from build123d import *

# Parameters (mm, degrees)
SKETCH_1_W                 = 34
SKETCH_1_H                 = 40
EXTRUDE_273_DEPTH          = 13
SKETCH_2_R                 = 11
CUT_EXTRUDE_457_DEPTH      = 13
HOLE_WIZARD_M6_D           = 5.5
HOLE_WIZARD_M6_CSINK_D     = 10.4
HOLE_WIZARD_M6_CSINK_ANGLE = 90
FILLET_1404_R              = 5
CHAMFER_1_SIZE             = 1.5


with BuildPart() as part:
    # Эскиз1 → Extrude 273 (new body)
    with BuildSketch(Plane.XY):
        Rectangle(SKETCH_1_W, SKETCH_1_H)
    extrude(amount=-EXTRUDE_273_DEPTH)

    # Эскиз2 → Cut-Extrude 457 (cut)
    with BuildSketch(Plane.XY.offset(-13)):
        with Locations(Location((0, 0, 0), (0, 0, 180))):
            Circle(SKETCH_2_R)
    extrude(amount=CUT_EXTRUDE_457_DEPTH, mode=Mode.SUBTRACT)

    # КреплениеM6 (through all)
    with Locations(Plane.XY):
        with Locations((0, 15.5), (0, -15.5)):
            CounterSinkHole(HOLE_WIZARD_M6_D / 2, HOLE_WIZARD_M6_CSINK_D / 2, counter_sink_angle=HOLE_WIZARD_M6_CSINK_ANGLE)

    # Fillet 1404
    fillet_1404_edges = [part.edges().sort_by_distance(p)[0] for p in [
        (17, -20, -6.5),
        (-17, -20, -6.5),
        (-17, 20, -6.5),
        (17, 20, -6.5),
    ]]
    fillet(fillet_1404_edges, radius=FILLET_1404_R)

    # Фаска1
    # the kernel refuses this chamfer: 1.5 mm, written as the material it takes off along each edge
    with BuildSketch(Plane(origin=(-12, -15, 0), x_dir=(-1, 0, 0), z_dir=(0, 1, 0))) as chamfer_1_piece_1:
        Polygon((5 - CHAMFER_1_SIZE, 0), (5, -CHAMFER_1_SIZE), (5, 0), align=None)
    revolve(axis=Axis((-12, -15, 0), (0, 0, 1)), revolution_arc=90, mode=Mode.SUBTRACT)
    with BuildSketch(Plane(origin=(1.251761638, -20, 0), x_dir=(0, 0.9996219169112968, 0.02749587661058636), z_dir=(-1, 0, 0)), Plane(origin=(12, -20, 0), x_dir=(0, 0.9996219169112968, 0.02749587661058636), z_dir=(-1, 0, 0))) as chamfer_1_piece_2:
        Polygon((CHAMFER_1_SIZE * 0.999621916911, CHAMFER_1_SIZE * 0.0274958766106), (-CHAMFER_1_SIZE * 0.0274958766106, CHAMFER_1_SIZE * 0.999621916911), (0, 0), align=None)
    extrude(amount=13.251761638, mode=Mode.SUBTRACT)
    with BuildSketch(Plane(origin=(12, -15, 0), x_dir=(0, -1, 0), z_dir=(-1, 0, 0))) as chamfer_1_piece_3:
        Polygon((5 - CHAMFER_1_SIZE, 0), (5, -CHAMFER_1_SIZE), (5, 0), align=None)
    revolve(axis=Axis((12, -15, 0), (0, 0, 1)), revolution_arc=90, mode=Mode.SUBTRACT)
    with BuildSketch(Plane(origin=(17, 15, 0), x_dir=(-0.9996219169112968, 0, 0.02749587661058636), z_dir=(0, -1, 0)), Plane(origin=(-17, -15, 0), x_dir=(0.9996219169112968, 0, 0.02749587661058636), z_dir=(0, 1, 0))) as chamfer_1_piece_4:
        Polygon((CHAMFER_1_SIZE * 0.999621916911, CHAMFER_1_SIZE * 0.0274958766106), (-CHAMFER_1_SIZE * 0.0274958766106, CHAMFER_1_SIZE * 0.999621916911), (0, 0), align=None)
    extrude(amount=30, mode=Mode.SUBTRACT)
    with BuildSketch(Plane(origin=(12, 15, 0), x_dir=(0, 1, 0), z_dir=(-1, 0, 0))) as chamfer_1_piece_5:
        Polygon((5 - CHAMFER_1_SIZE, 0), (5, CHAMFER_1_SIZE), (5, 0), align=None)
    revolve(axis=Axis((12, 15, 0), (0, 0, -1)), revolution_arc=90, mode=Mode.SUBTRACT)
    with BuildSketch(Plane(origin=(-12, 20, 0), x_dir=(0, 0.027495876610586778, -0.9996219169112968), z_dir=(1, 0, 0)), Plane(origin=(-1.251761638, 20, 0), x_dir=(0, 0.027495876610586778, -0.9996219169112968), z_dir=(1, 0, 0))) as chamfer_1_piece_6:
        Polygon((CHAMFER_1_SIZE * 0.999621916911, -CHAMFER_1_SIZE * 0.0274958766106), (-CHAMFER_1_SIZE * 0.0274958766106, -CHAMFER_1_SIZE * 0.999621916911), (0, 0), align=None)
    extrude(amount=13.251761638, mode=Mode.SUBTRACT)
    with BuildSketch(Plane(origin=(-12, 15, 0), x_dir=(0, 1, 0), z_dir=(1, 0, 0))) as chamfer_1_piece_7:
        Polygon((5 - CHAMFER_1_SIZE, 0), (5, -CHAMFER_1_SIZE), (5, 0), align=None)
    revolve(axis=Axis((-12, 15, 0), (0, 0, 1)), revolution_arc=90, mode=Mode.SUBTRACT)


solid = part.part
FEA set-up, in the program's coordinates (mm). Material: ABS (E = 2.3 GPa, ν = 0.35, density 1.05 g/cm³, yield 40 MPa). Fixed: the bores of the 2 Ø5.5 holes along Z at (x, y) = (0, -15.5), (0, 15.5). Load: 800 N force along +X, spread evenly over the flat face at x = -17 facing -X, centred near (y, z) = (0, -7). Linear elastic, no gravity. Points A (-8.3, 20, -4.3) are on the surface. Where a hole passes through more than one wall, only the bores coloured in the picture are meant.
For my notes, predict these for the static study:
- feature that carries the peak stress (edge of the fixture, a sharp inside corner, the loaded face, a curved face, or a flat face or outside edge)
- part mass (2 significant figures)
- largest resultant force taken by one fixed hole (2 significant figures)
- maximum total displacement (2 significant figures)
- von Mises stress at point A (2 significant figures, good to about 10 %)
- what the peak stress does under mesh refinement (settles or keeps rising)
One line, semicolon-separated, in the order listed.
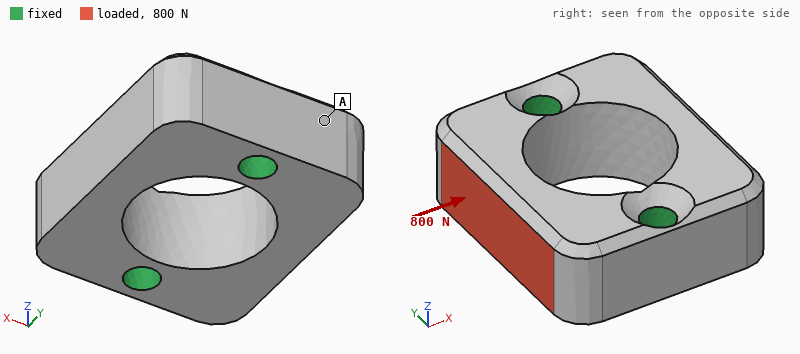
edge of the fixture; 12 g; 450 N; 68 µm; 1.1 MPa; keeps rising
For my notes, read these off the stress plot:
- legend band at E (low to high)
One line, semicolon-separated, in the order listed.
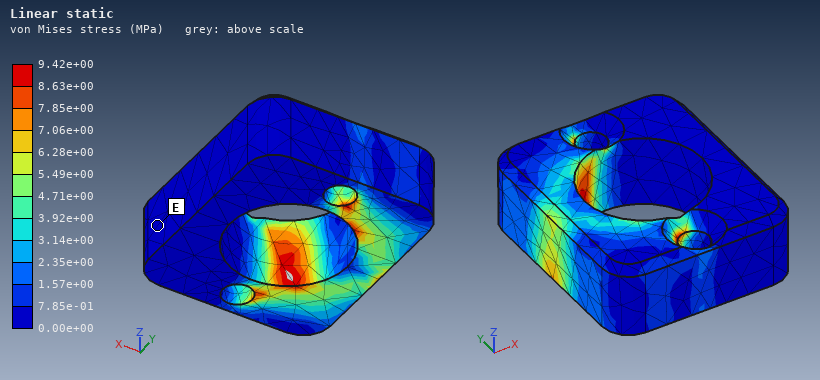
0.00e+00 to 7.85e-01 MPa
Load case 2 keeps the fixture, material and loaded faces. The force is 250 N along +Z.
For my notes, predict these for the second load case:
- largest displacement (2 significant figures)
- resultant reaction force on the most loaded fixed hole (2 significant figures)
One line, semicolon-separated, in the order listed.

0.10 mm; 130 N
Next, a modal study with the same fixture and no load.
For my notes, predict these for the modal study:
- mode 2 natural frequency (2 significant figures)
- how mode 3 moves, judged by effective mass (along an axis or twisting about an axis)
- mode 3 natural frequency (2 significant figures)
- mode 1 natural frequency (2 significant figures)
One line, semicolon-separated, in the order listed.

5800 Hz; twisting about Z; 7400 Hz; 5600 Hz
